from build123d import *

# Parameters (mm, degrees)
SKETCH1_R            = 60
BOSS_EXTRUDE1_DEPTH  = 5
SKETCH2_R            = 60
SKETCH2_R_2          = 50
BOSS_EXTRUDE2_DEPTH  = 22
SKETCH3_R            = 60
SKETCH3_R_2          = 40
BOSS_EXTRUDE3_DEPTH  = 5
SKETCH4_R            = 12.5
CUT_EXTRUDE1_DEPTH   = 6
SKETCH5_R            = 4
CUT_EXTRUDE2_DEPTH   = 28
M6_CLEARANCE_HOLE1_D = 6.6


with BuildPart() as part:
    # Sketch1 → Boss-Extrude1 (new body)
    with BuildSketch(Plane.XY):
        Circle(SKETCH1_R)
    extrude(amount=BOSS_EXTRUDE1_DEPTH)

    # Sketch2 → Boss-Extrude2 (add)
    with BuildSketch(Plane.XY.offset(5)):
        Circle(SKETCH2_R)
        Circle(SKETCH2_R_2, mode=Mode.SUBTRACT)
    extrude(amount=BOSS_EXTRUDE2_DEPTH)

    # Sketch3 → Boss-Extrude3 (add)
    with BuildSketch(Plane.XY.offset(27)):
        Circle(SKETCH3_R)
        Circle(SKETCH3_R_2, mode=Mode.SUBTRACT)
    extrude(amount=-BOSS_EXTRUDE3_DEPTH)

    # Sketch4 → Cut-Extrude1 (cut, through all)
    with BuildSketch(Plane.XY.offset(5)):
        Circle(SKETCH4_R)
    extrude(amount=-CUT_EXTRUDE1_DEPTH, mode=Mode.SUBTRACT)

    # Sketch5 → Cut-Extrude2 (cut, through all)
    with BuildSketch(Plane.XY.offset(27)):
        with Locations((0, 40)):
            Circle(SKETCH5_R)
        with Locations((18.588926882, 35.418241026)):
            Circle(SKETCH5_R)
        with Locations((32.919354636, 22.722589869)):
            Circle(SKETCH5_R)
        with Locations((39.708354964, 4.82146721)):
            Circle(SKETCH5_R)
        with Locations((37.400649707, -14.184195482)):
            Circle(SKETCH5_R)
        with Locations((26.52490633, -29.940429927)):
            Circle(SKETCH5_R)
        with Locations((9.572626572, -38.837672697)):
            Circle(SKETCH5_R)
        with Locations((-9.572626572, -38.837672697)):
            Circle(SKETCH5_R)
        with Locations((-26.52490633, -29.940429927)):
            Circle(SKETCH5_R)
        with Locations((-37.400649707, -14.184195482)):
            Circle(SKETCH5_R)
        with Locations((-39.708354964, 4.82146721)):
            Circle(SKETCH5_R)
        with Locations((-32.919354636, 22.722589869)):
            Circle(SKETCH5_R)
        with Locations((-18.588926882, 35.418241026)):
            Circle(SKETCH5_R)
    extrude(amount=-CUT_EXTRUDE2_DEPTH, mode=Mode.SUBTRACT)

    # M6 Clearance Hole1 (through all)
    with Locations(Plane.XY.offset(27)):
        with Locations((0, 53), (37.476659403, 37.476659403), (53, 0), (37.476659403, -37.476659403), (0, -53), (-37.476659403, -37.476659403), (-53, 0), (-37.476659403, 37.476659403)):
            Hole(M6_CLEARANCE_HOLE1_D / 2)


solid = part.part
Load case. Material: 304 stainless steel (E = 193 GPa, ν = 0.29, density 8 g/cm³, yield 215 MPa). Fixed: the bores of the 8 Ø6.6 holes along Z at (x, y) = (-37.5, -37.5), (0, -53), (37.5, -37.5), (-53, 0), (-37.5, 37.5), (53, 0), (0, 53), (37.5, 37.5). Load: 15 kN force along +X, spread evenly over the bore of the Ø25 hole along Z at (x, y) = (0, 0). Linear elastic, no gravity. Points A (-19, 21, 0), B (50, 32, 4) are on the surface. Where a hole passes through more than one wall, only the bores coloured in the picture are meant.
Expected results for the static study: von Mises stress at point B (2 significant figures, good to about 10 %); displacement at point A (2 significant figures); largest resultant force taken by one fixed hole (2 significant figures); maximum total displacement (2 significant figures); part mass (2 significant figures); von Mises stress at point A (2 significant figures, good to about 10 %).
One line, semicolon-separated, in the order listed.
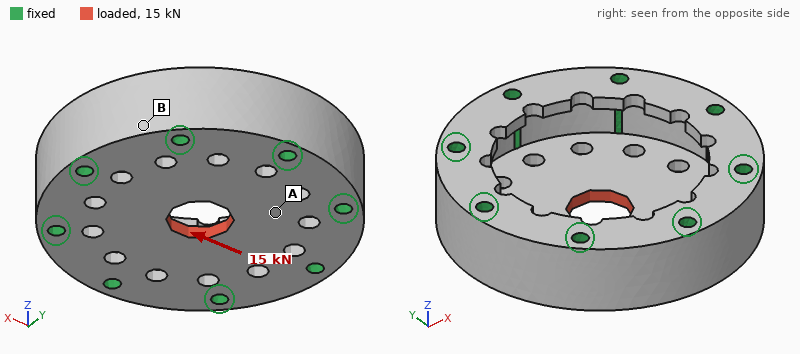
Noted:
7.1 MPa; 3.6 µm; 2.9 kN; 7.2 µm; 1.1 kg; 23 MPa
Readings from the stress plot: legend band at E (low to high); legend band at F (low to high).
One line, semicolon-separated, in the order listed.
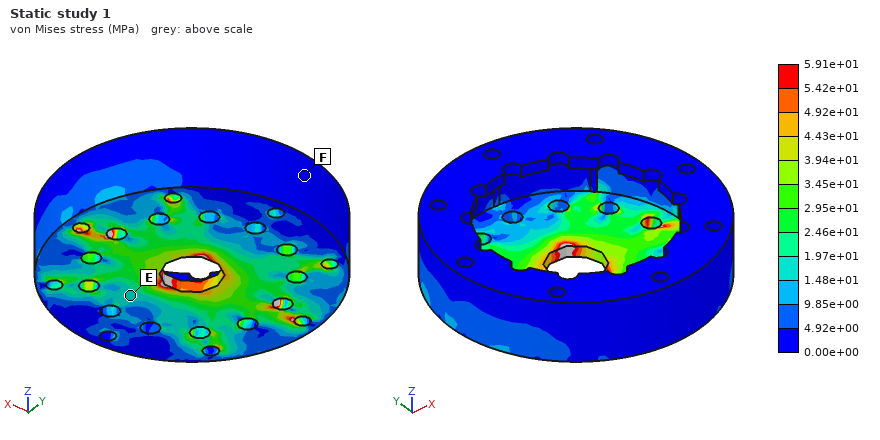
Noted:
1.48e+01 to 1.97e+01 MPa; 0.00e+00 to 4.92e+00 MPa
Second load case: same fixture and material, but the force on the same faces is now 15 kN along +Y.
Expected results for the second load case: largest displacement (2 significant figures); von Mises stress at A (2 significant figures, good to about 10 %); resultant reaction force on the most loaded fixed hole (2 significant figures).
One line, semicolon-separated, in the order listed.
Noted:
7.2 µm; 25 MPa; 3.0 kN
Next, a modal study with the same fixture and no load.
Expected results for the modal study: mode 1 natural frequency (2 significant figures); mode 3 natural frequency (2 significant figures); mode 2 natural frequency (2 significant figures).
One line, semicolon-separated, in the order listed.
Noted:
4300 Hz; 8100 Hz; 8100 Hz
